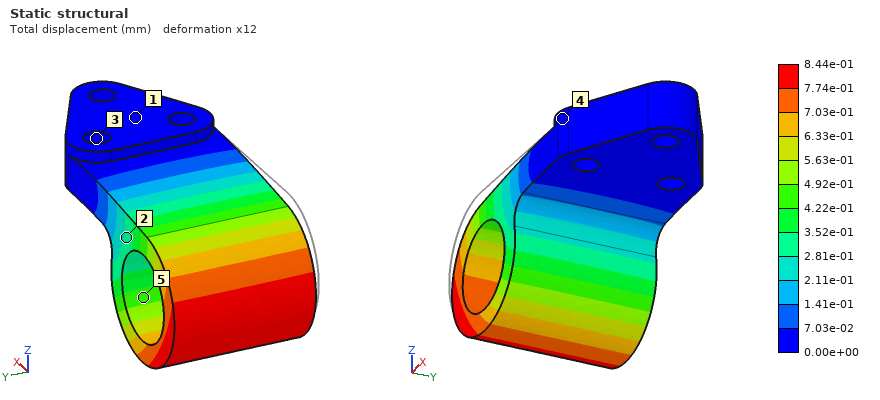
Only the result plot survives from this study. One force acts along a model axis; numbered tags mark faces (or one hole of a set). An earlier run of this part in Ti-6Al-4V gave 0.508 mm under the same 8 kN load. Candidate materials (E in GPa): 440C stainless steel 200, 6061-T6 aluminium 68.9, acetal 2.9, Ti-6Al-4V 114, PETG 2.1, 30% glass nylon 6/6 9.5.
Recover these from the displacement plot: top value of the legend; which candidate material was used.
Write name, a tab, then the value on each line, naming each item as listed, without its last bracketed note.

top value of the legend	8.44e-01 mm
which candidate material was used	6061-T6 aluminium
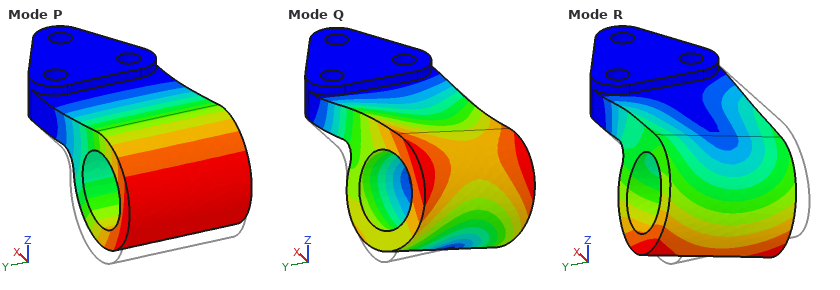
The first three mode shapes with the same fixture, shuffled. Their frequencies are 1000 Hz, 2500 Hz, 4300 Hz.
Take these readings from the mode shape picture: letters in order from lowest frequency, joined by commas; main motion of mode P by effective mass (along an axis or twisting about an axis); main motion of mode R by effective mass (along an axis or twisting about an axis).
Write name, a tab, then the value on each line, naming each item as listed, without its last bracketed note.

letters in order from lowest frequency, joined by commas	P, R, Q
main motion of mode P by effective mass	along Z
main motion of mode R by effective mass	along Y
